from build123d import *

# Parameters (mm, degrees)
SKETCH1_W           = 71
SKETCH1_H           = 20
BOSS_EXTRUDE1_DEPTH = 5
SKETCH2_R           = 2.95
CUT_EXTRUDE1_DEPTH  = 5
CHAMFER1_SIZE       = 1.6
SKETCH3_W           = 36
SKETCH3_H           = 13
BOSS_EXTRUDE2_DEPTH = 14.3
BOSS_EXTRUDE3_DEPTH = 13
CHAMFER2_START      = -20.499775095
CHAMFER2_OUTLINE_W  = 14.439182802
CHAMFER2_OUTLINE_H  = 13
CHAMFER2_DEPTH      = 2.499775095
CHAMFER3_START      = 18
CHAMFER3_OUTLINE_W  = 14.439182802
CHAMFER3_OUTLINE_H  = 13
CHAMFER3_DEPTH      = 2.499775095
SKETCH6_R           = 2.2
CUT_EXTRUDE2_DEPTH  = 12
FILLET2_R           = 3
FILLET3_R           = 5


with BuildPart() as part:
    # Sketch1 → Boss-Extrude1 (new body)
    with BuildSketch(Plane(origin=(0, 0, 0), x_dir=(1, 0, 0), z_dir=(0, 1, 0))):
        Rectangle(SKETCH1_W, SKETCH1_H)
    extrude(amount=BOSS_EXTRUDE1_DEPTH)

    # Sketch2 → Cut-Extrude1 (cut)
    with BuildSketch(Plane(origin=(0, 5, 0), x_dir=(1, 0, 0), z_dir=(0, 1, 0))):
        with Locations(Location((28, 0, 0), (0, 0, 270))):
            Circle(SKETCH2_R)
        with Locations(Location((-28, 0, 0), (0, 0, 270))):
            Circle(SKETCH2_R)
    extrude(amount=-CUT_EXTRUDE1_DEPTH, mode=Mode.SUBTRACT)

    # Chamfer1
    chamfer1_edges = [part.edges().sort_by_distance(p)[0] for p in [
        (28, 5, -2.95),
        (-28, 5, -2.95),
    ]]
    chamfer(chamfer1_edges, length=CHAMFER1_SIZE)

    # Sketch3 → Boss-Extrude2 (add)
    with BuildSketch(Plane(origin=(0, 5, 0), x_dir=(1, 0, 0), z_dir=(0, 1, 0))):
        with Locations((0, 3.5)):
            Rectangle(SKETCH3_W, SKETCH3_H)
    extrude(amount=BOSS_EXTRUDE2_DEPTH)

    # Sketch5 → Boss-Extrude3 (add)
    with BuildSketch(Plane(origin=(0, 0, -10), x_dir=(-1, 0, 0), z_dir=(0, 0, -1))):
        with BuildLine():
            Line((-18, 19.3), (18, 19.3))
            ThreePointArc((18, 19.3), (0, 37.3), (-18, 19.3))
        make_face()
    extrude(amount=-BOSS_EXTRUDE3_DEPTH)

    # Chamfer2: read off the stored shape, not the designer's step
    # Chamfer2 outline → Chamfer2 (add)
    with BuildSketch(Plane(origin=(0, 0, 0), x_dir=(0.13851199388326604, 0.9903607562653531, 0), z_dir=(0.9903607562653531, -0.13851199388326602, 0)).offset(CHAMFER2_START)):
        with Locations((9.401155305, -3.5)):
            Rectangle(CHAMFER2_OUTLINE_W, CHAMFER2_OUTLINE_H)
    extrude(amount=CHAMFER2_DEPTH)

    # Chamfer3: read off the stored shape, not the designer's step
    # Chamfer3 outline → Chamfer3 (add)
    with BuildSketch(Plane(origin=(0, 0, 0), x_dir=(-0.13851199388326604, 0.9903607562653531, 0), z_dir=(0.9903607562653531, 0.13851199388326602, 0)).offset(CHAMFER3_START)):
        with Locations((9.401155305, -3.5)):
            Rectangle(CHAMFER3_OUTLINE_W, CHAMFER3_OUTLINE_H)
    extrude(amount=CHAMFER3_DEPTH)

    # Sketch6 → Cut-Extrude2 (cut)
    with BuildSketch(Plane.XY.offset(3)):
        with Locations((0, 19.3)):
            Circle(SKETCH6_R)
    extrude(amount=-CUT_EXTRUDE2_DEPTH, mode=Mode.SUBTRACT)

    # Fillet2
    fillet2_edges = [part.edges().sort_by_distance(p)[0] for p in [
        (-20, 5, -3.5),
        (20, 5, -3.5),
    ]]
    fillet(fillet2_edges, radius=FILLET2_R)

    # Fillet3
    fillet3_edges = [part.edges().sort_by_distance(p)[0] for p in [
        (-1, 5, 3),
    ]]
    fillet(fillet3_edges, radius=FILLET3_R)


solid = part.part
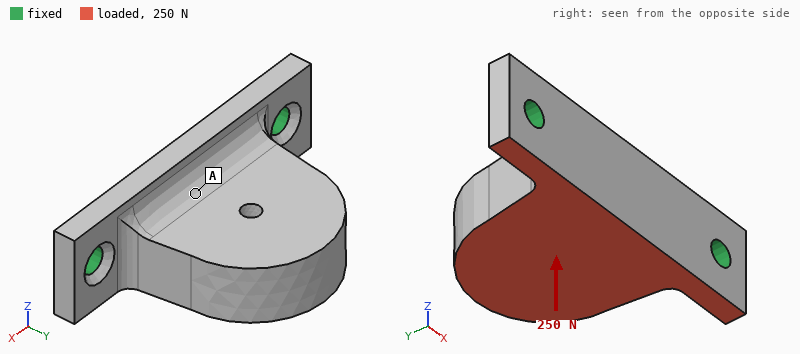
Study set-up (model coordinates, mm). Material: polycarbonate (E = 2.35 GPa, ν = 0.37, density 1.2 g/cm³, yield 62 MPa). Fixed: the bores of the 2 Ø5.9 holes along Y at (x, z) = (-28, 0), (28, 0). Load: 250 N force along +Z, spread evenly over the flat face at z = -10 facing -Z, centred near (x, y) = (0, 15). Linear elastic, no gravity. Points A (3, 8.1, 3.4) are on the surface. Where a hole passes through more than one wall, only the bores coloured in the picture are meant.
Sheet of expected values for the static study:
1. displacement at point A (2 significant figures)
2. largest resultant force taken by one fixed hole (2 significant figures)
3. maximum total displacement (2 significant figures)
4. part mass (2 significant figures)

0.18 mm
130 N
0.84 mm
25 g
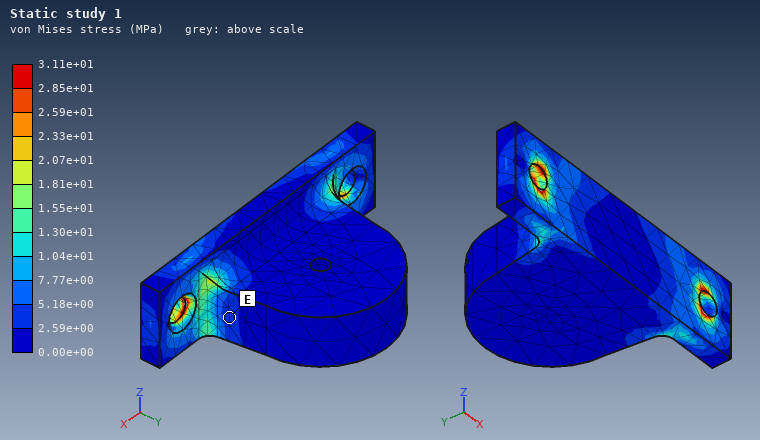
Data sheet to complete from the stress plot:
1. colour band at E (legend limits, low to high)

2.59e+00 to 5.18e+00 MPa
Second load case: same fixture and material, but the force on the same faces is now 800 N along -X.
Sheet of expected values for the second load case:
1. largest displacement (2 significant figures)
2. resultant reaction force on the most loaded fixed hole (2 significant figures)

0.15 mm
470 N
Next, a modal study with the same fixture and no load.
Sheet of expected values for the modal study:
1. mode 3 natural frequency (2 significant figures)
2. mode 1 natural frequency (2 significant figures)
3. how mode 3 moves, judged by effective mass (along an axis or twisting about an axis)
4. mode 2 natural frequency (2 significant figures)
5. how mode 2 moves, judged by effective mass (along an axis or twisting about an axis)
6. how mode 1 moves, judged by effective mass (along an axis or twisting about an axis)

2900 Hz
740 Hz
along X
2500 Hz
along Y
along Z
